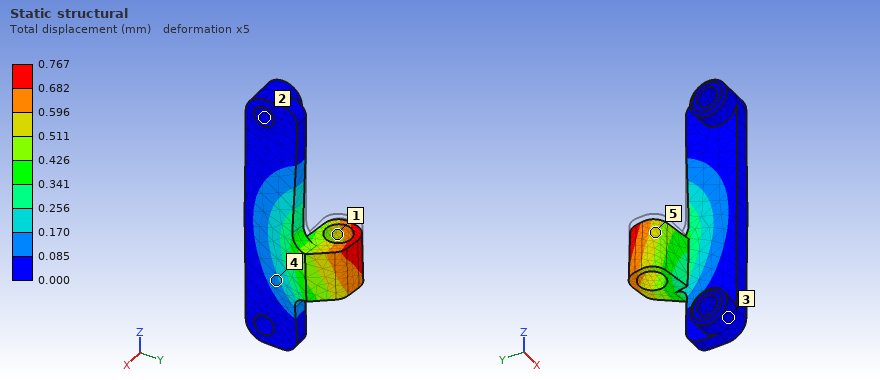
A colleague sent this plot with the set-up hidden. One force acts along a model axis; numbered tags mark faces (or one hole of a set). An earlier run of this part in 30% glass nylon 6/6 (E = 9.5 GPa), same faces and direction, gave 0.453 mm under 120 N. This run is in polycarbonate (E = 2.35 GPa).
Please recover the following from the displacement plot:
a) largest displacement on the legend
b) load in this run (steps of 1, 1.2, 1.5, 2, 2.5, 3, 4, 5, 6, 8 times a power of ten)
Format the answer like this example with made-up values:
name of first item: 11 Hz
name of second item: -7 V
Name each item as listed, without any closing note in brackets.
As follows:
largest displacement on the legend: 0.767 mm
load in this run: 50 N
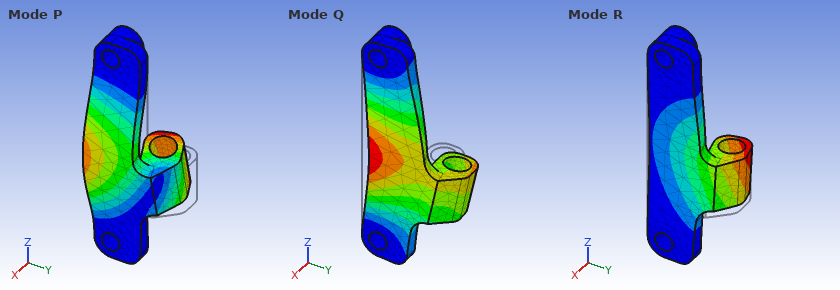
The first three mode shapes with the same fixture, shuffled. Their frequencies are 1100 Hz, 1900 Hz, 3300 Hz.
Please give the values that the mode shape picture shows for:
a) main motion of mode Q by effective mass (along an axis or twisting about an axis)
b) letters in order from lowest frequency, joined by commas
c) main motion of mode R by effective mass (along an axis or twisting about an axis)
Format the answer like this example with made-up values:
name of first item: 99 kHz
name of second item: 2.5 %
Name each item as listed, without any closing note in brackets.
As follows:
main motion of mode Q by effective mass: along Y
letters in order from lowest frequency, joined by commas: R, P, Q
main motion of mode R by effective mass: along X
